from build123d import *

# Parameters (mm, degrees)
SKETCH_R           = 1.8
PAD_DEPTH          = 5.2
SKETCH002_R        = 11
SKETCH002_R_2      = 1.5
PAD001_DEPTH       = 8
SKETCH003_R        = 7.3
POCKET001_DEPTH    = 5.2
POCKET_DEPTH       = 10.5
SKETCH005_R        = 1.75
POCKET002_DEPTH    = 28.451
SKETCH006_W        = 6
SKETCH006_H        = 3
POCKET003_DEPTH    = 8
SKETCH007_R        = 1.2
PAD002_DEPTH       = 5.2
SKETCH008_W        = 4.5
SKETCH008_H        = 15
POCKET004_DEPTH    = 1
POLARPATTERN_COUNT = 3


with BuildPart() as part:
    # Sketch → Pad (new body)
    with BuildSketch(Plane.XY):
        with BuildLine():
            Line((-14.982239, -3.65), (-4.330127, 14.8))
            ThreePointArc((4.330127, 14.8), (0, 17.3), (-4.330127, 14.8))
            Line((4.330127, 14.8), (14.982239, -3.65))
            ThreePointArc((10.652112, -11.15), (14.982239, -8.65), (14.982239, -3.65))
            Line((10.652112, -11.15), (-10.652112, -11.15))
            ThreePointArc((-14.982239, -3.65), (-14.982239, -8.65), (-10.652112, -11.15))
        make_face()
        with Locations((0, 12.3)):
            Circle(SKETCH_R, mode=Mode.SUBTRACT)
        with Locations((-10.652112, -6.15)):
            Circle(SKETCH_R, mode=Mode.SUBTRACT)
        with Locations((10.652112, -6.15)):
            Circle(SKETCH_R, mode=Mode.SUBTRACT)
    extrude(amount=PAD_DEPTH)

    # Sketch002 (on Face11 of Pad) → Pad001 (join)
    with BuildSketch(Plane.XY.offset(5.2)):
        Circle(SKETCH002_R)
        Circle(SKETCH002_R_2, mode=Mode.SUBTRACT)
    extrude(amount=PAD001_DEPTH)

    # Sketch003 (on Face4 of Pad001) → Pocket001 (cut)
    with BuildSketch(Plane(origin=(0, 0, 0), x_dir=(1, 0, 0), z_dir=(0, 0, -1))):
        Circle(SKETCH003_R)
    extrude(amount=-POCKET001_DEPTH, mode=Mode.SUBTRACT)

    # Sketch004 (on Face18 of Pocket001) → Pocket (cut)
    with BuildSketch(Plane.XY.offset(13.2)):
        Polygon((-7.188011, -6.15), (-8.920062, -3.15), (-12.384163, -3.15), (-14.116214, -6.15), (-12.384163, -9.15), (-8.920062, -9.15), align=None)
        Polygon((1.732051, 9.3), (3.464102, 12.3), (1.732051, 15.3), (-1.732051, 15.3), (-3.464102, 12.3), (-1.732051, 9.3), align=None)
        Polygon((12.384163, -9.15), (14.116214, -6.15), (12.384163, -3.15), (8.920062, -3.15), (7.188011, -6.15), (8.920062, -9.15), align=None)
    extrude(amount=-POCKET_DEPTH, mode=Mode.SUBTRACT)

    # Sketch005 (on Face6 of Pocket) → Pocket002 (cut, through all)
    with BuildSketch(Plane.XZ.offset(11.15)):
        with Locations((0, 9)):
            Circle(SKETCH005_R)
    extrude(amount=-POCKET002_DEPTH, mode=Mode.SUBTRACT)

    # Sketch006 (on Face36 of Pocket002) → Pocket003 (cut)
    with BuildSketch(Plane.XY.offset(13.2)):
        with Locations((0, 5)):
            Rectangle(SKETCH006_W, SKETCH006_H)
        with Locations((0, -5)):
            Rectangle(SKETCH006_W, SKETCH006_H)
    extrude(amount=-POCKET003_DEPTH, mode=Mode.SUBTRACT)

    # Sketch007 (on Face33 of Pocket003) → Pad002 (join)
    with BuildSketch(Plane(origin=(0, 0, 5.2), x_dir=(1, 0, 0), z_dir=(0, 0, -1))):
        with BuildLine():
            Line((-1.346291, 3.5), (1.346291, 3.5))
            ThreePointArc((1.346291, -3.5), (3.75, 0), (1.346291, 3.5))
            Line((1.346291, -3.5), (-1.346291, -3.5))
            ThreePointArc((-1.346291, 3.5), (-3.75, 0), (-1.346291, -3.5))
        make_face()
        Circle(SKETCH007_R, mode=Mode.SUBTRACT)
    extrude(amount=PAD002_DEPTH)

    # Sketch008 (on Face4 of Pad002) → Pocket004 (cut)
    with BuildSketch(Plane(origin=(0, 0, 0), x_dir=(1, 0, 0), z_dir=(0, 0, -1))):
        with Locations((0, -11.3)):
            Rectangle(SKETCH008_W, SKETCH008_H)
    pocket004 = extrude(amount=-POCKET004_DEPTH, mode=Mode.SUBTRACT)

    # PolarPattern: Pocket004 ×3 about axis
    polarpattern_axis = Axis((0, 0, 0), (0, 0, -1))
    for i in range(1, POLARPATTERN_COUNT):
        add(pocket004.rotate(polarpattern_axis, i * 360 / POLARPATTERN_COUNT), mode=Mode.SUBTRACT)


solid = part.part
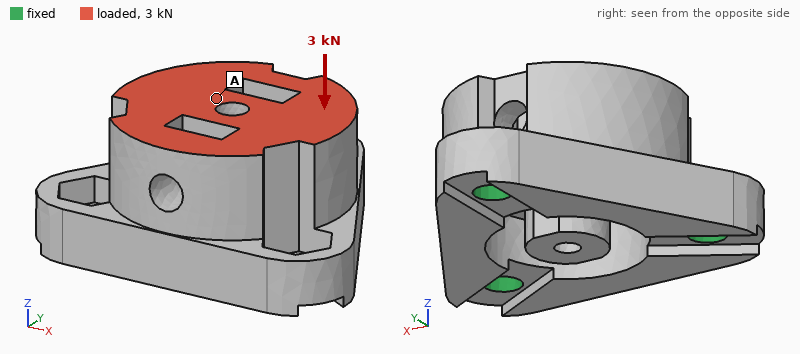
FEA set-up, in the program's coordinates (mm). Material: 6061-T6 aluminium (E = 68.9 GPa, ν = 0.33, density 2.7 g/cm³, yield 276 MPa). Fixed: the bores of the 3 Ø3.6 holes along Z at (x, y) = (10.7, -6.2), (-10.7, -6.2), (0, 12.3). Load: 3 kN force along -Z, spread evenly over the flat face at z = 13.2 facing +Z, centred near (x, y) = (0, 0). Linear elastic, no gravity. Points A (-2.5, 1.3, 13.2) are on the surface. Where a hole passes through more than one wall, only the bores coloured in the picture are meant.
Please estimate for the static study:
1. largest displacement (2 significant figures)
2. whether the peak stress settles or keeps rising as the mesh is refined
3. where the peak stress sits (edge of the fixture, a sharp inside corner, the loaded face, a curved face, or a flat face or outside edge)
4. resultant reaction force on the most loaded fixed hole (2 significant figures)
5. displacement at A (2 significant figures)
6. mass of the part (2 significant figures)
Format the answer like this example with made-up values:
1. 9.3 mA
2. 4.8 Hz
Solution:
1. 12 µm
2. keeps rising
3. edge of the fixture
4. 1.1 kN
5. 11 µm
6. 12 g
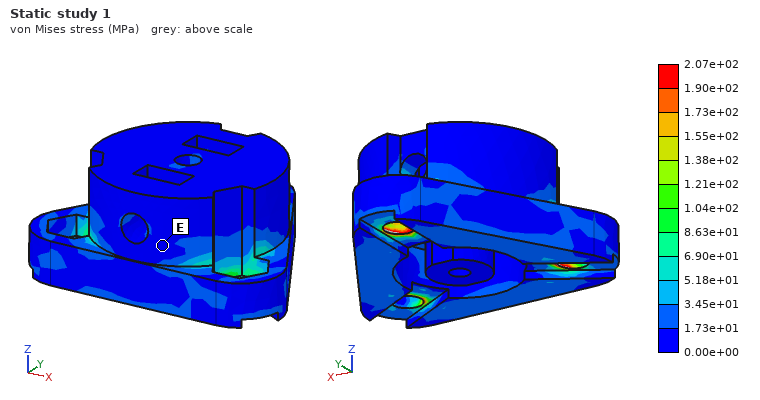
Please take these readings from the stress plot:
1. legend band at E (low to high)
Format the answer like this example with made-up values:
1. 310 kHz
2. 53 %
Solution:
1. 0.00e+00 to 1.73e+01 MPa
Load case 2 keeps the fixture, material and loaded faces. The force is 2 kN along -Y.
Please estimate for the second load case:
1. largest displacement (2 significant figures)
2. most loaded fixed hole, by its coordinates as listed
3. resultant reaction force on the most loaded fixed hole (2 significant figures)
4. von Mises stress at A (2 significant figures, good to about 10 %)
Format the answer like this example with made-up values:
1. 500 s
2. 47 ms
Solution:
1. 25 µm
2. (0, 12.3)
3. 1.5 kN
4. 21 MPa
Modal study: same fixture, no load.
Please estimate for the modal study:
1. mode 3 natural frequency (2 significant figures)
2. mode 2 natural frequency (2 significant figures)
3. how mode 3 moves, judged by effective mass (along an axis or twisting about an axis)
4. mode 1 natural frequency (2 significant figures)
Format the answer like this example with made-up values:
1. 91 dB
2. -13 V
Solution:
1. 27 kHz
2. 24 kHz
3. along Z
4. 23 kHz
